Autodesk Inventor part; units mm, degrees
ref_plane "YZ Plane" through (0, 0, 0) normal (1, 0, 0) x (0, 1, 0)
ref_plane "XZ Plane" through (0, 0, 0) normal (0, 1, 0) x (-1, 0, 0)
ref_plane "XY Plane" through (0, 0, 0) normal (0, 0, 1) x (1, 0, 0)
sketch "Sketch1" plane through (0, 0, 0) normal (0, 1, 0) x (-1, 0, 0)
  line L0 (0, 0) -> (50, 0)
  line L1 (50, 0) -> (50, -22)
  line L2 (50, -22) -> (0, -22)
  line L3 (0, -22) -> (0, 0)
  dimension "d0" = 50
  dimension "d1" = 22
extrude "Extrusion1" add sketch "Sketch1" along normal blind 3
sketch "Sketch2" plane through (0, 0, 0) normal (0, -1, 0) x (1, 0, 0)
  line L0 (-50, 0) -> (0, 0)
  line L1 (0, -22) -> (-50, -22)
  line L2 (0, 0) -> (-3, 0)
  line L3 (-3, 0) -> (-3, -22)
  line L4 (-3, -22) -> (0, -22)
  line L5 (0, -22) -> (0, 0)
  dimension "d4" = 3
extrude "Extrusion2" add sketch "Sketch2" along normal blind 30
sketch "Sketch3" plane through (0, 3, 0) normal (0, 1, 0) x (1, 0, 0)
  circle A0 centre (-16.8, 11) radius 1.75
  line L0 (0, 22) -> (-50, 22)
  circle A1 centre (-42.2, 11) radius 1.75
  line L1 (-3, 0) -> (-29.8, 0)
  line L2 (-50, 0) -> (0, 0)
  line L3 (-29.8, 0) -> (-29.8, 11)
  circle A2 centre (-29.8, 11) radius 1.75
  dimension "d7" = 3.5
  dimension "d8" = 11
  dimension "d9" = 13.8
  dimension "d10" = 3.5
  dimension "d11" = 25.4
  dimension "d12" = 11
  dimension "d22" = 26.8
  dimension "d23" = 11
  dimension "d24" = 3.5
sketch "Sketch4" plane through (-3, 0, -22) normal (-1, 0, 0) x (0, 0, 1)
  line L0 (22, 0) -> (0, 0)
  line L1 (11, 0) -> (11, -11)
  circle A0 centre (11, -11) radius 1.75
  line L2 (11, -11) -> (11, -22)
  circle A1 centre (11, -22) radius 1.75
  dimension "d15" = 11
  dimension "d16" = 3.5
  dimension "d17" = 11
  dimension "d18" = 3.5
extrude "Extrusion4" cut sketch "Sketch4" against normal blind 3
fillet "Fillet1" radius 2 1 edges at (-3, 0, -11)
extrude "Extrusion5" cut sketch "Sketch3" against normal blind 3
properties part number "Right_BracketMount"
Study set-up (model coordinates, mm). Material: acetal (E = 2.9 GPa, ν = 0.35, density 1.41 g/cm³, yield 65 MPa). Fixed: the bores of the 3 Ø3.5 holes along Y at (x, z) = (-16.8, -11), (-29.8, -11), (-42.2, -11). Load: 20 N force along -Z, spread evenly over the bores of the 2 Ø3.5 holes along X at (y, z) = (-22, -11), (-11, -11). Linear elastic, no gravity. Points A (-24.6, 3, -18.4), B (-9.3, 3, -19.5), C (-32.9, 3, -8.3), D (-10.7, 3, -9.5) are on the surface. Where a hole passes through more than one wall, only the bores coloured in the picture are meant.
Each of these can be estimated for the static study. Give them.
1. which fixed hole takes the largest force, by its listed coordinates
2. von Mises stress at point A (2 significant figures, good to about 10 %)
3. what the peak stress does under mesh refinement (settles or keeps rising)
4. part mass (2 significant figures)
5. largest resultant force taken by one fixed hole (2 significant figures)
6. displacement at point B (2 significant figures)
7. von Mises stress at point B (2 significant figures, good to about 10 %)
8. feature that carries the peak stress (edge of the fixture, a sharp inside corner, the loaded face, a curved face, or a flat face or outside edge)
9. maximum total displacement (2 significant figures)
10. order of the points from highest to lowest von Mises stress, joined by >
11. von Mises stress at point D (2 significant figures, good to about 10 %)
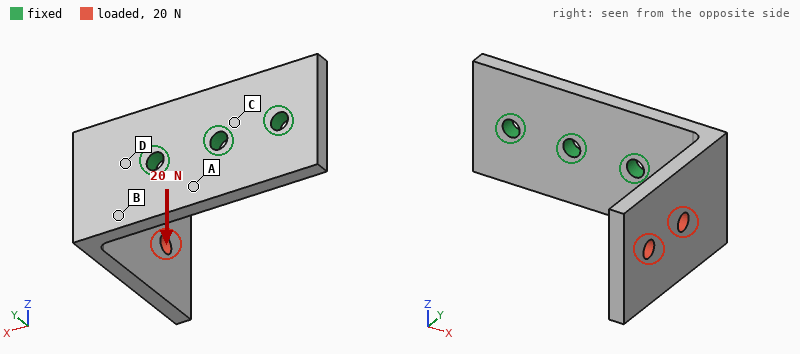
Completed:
(-16.8, -11)
2.8 MPa
keeps rising
7.3 g
33 N
0.12 mm
5.2 MPa
edge of the fixture
0.73 mm
D > B > A > C
7.3 MPa
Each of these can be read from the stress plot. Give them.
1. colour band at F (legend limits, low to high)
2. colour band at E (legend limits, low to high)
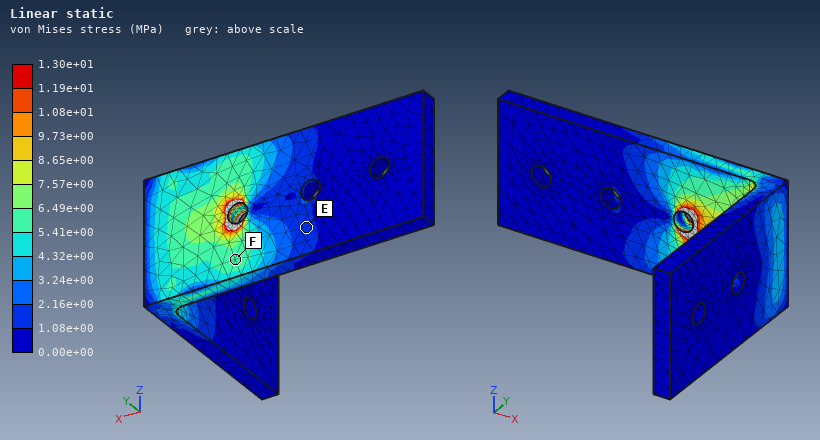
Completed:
5.41e+00 to 6.49e+00 MPa
1.08e+00 to 2.16e+00 MPa
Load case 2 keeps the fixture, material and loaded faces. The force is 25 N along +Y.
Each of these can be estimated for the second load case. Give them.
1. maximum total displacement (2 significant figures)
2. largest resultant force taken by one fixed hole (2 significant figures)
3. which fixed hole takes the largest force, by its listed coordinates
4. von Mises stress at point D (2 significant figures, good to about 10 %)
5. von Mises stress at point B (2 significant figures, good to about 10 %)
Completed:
0.67 mm
35 N
(-16.8, -11)
7.0 MPa
5.3 MPa
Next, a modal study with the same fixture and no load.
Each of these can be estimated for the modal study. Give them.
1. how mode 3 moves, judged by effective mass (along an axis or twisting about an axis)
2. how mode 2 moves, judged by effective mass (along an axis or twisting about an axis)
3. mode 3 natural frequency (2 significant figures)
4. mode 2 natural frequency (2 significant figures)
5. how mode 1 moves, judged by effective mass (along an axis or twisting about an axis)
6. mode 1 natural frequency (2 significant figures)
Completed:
along Y
along Z
1400 Hz
620 Hz
along X
420 Hz
